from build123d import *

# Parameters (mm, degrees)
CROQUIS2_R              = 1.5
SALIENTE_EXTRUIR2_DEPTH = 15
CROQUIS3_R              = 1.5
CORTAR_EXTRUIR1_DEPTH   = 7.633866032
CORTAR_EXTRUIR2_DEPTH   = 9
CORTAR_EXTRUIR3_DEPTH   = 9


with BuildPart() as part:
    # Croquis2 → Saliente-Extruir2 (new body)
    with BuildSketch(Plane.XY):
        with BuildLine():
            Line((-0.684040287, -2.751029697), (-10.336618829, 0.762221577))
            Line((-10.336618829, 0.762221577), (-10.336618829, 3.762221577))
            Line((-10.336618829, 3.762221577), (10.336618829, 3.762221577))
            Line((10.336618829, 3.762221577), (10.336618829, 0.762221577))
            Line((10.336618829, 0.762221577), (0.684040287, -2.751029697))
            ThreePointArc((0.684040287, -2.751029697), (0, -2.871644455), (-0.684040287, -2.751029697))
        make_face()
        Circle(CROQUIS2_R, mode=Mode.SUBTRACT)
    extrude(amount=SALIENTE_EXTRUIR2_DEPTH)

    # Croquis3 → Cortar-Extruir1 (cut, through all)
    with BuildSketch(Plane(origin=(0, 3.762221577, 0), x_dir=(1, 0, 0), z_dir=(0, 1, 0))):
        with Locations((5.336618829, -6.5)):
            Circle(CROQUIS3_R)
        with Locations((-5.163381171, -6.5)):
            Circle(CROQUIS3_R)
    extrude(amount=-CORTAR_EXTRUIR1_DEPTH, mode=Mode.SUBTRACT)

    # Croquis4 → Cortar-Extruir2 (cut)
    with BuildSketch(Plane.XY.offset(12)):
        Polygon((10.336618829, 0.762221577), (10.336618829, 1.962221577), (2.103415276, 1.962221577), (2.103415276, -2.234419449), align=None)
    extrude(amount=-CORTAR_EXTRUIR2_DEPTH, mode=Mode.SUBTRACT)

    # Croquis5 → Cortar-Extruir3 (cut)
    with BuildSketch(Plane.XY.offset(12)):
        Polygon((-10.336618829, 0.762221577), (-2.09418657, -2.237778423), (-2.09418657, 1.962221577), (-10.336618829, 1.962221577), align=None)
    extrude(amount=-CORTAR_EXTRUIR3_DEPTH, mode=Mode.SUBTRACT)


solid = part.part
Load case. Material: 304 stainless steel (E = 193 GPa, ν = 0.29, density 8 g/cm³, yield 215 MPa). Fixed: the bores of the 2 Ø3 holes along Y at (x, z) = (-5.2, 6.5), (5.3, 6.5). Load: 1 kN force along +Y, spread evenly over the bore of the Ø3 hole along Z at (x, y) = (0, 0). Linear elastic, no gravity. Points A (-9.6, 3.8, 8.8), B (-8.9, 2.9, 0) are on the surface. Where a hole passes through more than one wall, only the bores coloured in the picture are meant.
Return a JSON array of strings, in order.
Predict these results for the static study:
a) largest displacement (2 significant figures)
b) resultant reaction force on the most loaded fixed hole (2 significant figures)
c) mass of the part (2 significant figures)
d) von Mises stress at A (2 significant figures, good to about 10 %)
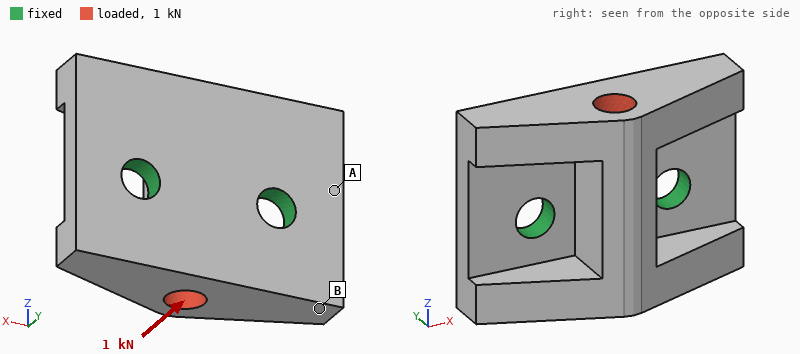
["8.6 µm", "530 N", "7.8 g", "38 MPa"]
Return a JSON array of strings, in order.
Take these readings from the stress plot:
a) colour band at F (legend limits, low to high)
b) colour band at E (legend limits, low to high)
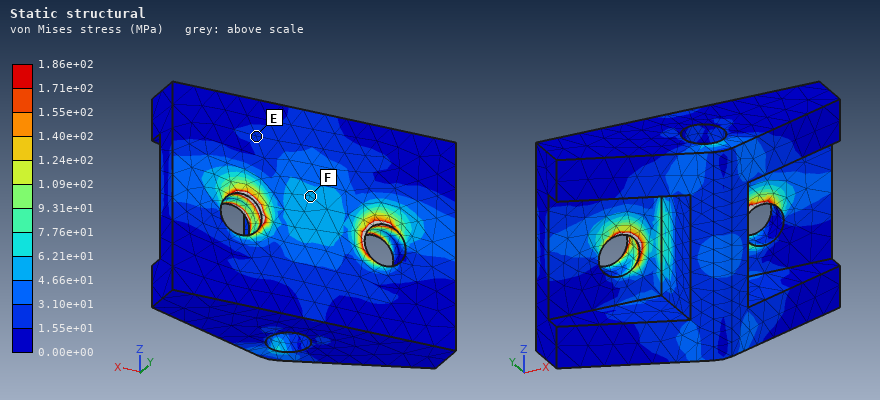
["4.66e+01 to 6.21e+01 MPa", "1.55e+01 to 3.10e+01 MPa"]
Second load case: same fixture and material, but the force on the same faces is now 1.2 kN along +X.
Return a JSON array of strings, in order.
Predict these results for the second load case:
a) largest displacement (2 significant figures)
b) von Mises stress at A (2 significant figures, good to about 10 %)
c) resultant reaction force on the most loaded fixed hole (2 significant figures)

["6.4 µm", "42 MPa", "690 N"]
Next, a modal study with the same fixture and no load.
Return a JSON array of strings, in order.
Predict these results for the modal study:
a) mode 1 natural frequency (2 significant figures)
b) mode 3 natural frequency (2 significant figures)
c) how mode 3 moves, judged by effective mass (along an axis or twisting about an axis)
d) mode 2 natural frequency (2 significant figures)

["17 kHz", "36 kHz", "along Y", "28 kHz"]
